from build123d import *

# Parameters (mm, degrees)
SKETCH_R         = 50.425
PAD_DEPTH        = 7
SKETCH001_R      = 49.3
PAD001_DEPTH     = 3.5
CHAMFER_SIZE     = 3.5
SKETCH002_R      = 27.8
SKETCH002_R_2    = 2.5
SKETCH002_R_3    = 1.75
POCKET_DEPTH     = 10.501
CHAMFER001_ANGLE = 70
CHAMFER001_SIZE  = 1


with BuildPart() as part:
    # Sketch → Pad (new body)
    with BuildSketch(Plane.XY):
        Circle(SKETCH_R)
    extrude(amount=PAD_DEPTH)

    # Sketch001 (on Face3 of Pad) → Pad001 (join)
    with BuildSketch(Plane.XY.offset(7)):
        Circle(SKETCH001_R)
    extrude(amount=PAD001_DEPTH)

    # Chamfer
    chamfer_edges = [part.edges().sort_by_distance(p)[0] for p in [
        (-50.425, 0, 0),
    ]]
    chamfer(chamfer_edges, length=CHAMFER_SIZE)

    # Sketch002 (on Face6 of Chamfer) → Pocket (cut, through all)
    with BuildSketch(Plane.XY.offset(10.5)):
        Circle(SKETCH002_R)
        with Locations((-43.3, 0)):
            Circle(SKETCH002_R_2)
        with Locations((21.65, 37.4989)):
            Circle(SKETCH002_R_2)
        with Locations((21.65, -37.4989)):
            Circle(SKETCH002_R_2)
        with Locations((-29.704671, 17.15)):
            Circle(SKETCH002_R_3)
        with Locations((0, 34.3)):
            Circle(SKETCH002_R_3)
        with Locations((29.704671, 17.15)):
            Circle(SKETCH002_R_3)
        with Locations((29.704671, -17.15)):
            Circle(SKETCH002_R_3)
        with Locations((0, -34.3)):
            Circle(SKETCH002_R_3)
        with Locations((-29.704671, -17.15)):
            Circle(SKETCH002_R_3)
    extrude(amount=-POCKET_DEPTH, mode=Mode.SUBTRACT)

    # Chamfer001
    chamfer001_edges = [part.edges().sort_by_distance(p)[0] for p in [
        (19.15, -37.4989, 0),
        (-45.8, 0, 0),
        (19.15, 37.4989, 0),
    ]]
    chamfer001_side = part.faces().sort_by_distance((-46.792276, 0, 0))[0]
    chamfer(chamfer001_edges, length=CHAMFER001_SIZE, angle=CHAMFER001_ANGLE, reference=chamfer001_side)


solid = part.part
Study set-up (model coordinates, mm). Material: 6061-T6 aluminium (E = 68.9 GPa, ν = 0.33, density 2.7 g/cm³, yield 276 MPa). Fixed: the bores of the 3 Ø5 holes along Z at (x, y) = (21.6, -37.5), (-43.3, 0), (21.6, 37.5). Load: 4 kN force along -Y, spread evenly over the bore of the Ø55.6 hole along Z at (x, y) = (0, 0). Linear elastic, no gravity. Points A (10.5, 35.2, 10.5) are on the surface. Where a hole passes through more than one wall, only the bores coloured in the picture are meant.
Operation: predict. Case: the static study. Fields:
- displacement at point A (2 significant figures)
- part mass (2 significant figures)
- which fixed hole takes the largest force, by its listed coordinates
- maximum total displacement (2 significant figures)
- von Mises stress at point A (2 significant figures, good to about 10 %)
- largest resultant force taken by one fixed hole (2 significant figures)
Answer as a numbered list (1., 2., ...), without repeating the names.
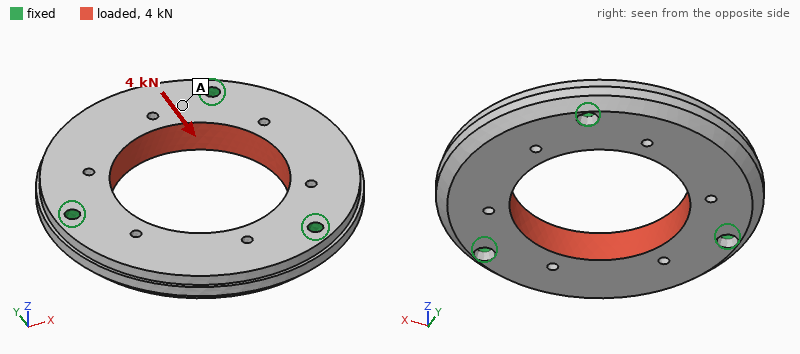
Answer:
1. 1.7 µm
2. 150 g
3. (-43.3, 0)
4. 4.9 µm
5. 3.3 MPa
6. 1.7 kN
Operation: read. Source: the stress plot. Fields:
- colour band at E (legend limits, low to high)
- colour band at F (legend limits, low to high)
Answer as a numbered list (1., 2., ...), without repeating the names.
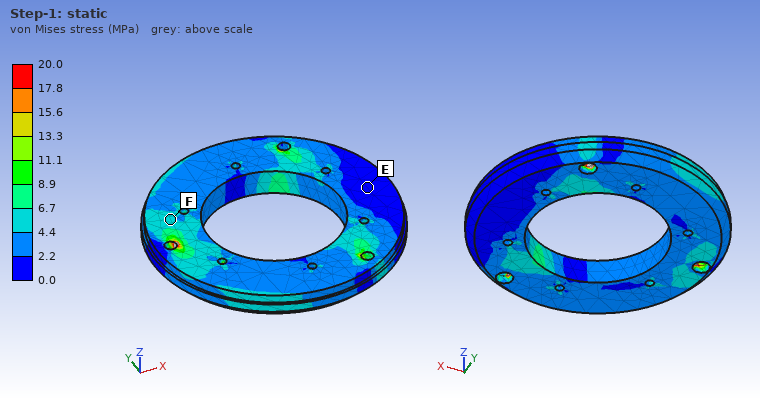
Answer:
1. 0.0 to 2.2 MPa
2. 4.4 to 6.7 MPa
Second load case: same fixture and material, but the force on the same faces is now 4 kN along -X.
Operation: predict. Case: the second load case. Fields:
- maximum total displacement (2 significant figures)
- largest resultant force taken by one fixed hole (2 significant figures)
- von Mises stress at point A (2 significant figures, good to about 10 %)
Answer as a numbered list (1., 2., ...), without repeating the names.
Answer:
1. 5.6 µm
2. 1.6 kN
3. 6.9 MPa
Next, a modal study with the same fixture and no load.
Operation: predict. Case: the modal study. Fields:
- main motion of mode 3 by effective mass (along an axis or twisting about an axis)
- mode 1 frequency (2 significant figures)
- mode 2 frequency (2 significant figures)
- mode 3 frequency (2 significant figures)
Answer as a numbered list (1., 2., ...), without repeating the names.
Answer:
1. along Z
2. 5100 Hz
3. 5100 Hz
4. 6100 Hz
